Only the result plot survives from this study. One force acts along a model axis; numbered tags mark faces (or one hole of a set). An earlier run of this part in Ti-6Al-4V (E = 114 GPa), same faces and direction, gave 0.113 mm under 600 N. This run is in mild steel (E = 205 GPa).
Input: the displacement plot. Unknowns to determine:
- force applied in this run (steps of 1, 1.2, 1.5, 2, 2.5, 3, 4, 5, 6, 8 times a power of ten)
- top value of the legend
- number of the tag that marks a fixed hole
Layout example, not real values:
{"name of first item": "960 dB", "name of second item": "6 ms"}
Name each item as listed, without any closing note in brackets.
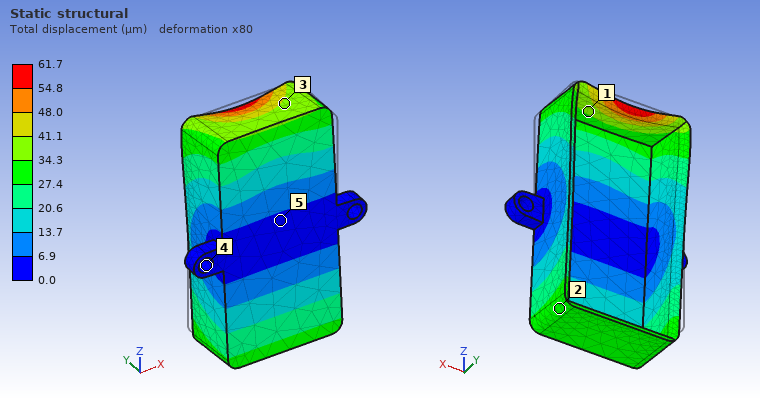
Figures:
{"force applied in this run": "600 N", "top value of the legend": "61.7 µm", "number of the tag that marks a fixed hole": "4"}
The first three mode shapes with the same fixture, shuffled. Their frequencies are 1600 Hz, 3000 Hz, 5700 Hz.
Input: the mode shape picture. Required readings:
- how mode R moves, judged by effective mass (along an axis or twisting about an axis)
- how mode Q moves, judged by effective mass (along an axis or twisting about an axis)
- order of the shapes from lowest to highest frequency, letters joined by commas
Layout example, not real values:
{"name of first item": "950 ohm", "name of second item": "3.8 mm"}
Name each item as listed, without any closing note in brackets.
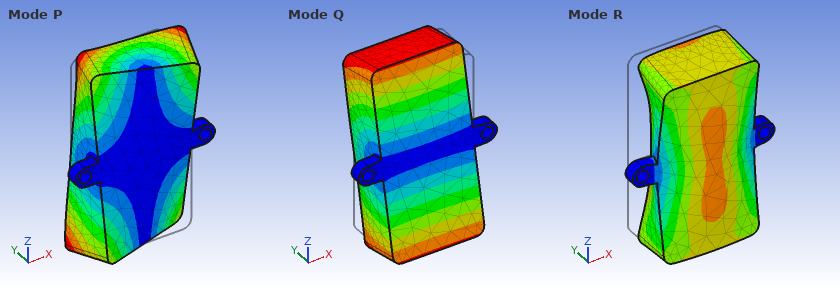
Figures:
{"how mode R moves, judged by effective mass": "along Y", "how mode Q moves, judged by effective mass": "twisting about X", "order of the shapes from lowest to highest frequency, letters joined by commas": "Q, P, R"}
